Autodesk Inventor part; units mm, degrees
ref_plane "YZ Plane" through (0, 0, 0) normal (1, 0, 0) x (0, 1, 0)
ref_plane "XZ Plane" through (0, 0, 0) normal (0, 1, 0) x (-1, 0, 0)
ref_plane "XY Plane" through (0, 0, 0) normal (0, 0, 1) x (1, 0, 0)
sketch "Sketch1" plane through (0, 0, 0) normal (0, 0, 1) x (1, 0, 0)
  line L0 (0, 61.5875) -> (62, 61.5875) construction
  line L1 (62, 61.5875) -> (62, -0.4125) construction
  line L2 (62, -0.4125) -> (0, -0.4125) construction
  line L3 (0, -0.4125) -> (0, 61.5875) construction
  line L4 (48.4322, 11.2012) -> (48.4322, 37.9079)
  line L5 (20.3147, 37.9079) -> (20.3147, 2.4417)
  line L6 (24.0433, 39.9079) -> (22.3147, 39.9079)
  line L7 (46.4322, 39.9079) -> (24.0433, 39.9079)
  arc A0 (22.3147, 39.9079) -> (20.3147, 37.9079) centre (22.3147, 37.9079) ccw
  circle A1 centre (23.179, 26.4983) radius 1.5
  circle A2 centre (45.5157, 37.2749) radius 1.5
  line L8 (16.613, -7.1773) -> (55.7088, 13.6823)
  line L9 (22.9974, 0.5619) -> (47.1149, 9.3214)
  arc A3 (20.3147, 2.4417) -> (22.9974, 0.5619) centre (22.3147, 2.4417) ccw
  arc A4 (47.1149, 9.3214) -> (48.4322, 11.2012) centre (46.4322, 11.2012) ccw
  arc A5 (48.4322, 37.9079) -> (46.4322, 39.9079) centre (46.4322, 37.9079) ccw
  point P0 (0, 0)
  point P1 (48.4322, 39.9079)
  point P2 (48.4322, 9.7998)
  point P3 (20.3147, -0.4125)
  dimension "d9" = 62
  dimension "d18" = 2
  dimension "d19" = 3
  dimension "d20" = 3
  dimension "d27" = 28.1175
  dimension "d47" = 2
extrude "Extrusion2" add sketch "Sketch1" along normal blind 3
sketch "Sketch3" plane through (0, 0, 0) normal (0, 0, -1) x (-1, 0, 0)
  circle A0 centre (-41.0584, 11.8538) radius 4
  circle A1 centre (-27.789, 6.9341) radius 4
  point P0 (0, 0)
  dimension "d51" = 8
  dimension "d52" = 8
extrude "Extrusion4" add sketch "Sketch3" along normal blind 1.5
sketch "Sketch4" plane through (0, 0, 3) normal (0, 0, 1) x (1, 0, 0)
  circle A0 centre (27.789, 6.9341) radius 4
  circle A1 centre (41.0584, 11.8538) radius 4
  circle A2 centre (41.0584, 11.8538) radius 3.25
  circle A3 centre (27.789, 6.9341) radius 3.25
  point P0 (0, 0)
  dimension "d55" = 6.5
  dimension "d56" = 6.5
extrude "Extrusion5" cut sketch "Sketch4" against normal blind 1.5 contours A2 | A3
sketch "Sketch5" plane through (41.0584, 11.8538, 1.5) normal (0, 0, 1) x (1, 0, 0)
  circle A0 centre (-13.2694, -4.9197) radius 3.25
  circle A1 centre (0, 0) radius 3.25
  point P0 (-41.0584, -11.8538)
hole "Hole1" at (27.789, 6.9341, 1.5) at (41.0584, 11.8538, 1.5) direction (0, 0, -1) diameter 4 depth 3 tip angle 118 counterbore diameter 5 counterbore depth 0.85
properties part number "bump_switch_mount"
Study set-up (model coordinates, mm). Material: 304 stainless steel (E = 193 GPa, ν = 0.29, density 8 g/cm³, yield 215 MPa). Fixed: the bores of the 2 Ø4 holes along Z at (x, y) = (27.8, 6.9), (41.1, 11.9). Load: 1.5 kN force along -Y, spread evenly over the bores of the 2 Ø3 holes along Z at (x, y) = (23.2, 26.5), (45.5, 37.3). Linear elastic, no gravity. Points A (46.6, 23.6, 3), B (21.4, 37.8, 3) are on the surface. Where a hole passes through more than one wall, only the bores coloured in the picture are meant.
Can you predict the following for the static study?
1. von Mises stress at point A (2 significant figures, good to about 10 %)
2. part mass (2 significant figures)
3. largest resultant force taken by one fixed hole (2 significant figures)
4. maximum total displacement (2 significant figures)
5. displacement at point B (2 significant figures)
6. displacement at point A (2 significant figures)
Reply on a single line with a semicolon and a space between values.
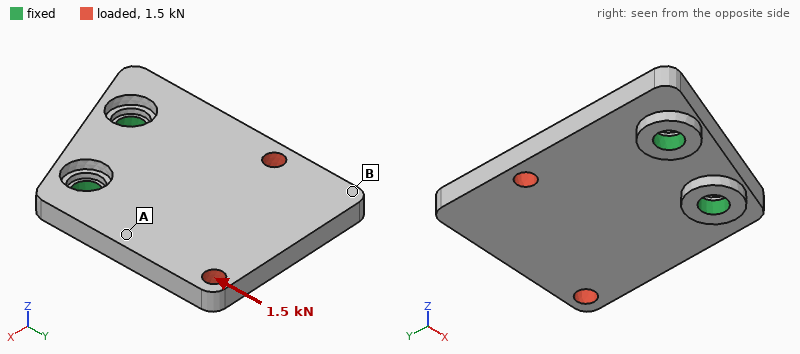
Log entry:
23 MPa; 23 g; 760 N; 19 µm; 18 µm; 6.9 µm
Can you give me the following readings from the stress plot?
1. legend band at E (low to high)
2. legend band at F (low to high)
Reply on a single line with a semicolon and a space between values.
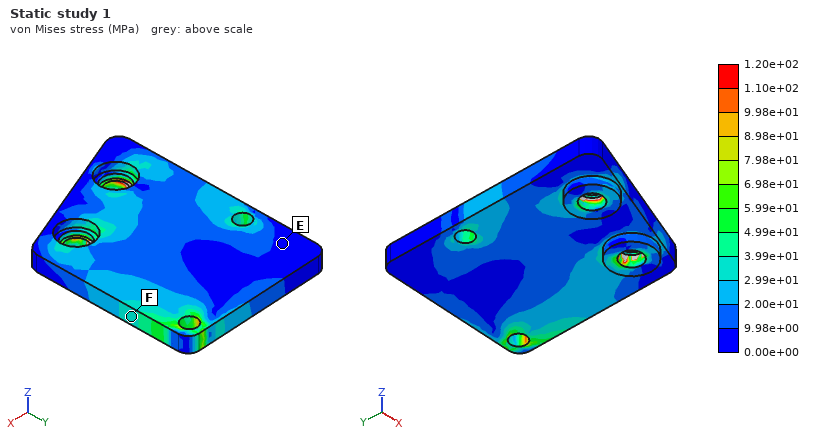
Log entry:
0.00e+00 to 9.98e+00 MPa; 2.99e+01 to 3.99e+01 MPa
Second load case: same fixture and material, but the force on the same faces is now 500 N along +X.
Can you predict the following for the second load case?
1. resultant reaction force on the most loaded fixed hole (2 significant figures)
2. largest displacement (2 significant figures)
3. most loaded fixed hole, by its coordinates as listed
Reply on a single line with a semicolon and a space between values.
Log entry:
720 N; 12 µm; (41.1, 11.9)
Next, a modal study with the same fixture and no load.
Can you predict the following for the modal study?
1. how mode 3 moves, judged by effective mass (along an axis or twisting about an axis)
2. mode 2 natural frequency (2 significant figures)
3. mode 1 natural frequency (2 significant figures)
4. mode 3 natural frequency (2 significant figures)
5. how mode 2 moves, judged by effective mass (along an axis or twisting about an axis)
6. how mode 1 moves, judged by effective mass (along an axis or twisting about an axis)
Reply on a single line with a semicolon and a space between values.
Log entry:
along X; 6400 Hz; 2600 Hz; 12 kHz; twisting about Y; along Z
